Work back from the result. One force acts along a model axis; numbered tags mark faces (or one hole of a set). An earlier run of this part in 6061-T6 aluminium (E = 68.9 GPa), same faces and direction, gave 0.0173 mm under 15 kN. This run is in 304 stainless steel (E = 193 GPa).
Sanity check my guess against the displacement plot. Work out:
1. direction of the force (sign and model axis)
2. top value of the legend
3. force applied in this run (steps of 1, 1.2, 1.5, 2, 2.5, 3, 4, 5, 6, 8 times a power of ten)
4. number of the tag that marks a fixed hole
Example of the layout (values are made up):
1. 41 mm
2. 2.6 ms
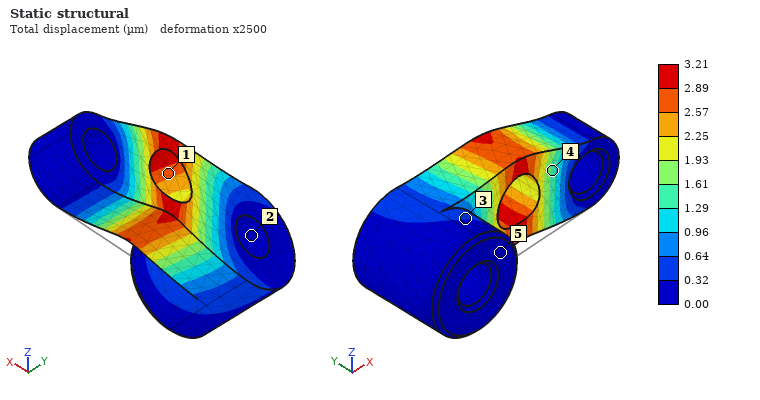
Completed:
1. +Z
2. 3.21 µm
3. 8 kN
4. 2
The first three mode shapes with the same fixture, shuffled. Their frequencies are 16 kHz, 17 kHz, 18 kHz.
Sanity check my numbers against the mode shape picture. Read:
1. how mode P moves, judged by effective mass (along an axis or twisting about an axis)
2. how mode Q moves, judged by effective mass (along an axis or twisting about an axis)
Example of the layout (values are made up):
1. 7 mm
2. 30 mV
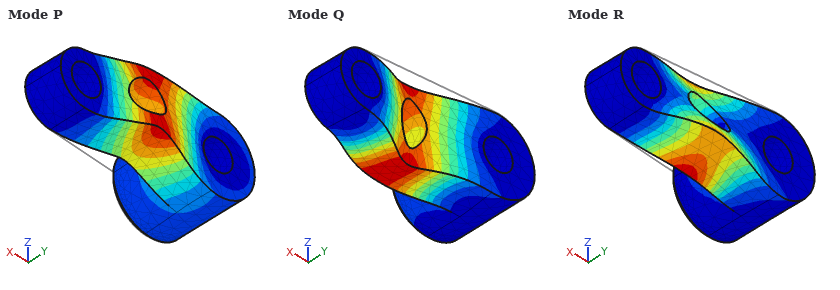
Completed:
1. along Z
2. along Y
